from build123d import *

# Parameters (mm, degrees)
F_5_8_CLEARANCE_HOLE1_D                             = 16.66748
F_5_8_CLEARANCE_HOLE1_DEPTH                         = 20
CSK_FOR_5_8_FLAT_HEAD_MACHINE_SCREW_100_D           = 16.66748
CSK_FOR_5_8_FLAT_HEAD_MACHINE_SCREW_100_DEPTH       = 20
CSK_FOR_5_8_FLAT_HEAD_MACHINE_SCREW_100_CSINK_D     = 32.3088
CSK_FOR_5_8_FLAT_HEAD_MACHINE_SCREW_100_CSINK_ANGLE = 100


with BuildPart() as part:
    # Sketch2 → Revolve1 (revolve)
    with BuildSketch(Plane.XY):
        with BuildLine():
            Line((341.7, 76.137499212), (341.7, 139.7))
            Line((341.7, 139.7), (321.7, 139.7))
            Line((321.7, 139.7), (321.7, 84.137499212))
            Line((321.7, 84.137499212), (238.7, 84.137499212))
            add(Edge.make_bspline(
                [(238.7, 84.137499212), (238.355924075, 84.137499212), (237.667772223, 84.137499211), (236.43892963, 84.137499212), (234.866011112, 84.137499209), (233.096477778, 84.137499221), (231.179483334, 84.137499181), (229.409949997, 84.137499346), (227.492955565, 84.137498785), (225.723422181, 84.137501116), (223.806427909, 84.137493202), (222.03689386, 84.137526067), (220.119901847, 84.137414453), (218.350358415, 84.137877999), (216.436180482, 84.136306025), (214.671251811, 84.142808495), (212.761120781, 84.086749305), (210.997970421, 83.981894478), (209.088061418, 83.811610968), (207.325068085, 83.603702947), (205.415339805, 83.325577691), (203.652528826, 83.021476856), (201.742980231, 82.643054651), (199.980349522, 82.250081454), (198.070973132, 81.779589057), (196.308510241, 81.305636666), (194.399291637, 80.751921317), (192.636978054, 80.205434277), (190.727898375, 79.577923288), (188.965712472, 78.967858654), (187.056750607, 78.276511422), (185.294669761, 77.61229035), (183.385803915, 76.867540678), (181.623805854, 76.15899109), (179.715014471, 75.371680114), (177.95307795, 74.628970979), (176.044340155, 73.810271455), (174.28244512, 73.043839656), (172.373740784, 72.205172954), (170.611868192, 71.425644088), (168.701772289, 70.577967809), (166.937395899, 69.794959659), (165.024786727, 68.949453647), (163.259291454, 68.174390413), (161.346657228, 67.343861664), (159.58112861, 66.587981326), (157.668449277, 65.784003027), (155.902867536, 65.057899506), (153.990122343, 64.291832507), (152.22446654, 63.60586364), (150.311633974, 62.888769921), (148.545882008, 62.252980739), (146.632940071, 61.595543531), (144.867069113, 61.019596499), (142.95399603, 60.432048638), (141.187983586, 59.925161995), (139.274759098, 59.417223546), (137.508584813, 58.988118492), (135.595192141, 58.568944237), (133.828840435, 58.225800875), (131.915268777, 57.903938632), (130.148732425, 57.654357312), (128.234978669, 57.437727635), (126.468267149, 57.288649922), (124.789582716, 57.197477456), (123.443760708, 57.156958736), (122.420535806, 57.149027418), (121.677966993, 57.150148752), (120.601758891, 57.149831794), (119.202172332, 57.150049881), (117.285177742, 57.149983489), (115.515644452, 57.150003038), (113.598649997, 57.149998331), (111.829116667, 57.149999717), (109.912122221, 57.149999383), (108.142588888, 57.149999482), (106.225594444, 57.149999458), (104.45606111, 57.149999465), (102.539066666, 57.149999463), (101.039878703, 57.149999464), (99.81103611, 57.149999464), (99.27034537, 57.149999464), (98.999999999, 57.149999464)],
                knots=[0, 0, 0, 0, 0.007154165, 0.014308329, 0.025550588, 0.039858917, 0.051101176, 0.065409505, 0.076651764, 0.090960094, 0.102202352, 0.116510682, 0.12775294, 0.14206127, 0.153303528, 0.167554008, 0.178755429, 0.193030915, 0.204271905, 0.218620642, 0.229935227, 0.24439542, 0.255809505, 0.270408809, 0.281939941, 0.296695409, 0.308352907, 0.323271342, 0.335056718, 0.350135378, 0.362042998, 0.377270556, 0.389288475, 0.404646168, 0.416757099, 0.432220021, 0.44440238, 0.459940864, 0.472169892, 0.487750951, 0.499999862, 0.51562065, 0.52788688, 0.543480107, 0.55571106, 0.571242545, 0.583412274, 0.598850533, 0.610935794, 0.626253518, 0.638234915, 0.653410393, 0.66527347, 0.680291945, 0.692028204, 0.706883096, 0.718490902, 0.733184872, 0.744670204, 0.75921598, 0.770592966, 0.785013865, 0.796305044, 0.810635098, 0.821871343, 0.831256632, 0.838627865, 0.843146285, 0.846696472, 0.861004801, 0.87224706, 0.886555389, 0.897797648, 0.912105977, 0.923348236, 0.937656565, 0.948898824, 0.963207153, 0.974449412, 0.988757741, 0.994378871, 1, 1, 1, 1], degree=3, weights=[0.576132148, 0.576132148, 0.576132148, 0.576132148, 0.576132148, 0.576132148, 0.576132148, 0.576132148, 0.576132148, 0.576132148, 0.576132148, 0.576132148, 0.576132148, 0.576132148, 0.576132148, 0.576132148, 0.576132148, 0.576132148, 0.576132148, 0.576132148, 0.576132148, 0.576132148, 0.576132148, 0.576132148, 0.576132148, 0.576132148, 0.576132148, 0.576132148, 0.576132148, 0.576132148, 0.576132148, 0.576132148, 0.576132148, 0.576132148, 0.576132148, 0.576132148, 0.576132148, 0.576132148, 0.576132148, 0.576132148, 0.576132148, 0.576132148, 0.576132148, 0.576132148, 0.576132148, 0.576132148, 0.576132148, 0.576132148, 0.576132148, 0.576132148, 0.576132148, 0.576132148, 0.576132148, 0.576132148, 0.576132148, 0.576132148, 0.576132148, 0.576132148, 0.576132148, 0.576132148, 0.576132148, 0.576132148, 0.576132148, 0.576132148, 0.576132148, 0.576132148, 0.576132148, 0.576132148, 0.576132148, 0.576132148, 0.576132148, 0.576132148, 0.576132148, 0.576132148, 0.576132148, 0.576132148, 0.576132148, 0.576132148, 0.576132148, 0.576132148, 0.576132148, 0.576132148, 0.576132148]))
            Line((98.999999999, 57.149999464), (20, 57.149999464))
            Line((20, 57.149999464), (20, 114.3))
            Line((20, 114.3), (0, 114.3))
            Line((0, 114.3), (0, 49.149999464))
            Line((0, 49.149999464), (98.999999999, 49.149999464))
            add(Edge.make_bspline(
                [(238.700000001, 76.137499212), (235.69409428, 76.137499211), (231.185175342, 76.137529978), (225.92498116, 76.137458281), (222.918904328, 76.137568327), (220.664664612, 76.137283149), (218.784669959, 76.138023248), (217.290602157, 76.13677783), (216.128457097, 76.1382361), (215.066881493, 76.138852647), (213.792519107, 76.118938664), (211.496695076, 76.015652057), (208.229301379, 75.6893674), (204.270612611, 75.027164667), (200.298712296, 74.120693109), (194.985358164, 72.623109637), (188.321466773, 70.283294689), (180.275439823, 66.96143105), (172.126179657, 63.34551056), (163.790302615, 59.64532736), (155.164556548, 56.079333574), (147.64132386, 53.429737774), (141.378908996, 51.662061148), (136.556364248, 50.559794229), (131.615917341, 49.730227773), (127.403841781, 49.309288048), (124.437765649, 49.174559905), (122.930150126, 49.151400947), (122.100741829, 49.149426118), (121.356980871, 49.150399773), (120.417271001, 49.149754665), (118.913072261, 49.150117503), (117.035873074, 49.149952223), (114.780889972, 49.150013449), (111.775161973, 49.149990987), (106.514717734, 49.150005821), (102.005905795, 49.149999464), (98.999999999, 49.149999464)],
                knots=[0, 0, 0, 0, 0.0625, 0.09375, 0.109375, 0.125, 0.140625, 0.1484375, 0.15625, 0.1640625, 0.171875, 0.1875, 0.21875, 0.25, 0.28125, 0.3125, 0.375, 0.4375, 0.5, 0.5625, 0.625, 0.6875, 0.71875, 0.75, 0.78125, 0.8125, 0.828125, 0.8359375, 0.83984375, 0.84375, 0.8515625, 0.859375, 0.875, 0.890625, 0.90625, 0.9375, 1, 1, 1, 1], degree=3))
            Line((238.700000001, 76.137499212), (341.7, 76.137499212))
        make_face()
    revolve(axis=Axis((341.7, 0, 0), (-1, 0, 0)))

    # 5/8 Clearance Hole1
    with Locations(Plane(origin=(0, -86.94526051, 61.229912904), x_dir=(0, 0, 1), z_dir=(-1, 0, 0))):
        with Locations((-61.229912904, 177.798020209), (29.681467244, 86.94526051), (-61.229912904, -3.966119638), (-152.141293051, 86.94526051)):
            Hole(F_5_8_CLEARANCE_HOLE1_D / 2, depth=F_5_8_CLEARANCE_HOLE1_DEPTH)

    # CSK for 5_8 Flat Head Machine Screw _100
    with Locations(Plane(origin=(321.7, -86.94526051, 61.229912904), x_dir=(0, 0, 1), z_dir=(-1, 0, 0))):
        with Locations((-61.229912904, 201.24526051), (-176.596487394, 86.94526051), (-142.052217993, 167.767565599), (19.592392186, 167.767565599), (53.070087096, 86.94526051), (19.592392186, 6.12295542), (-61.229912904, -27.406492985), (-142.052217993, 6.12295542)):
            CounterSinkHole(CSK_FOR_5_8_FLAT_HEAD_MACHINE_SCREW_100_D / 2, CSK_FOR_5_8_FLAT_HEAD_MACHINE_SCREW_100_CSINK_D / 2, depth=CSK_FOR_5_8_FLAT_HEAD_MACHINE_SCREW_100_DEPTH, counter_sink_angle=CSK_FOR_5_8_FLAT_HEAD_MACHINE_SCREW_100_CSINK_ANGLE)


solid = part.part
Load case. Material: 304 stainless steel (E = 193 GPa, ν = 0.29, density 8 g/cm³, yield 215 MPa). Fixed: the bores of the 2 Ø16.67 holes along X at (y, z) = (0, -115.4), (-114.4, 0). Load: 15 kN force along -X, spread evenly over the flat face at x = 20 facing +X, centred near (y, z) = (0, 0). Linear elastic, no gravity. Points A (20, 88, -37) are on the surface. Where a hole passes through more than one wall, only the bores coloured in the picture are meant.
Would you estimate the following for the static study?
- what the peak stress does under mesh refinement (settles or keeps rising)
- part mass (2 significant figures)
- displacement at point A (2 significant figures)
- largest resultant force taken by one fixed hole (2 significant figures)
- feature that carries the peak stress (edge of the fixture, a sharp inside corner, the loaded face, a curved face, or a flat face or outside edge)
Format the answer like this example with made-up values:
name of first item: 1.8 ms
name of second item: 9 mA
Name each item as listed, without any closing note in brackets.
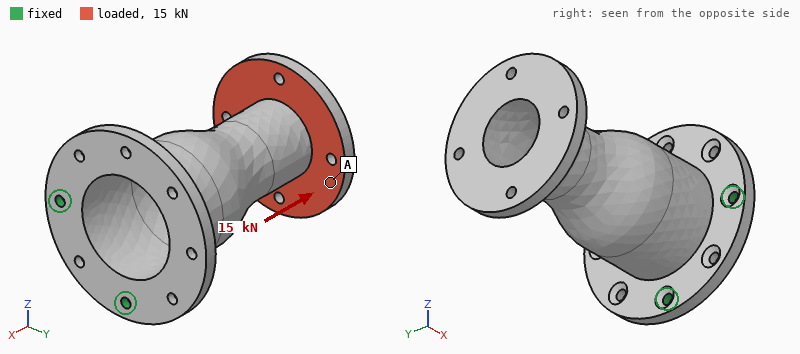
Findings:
what the peak stress does under mesh refinement: keeps rising
part mass: 20 kg
displacement at point A: 0.77 mm
largest resultant force taken by one fixed hole: 7.5 kN
feature that carries the peak stress: edge of the fixture
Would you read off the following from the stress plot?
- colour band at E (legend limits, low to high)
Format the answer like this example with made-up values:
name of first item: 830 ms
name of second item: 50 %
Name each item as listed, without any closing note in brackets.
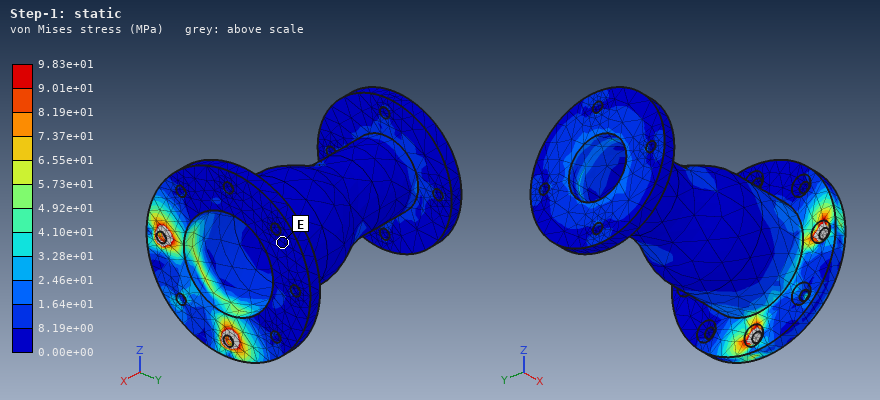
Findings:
colour band at E: 0.00e+00 to 8.19e+00 MPa
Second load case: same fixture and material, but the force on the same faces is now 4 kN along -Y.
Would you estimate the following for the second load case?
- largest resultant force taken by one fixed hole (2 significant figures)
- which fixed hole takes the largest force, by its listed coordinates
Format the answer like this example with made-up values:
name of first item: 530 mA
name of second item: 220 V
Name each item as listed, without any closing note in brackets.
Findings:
largest resultant force taken by one fixed hole: 7.7 kN
which fixed hole takes the largest force, by its listed coordinates: (-114.4, 0)
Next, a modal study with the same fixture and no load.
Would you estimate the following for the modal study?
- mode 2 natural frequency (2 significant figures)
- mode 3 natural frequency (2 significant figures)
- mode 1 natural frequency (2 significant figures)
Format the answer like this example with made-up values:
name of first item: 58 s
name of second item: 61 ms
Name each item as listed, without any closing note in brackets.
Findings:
mode 2 natural frequency: 310 Hz
mode 3 natural frequency: 910 Hz
mode 1 natural frequency: 110 Hz
